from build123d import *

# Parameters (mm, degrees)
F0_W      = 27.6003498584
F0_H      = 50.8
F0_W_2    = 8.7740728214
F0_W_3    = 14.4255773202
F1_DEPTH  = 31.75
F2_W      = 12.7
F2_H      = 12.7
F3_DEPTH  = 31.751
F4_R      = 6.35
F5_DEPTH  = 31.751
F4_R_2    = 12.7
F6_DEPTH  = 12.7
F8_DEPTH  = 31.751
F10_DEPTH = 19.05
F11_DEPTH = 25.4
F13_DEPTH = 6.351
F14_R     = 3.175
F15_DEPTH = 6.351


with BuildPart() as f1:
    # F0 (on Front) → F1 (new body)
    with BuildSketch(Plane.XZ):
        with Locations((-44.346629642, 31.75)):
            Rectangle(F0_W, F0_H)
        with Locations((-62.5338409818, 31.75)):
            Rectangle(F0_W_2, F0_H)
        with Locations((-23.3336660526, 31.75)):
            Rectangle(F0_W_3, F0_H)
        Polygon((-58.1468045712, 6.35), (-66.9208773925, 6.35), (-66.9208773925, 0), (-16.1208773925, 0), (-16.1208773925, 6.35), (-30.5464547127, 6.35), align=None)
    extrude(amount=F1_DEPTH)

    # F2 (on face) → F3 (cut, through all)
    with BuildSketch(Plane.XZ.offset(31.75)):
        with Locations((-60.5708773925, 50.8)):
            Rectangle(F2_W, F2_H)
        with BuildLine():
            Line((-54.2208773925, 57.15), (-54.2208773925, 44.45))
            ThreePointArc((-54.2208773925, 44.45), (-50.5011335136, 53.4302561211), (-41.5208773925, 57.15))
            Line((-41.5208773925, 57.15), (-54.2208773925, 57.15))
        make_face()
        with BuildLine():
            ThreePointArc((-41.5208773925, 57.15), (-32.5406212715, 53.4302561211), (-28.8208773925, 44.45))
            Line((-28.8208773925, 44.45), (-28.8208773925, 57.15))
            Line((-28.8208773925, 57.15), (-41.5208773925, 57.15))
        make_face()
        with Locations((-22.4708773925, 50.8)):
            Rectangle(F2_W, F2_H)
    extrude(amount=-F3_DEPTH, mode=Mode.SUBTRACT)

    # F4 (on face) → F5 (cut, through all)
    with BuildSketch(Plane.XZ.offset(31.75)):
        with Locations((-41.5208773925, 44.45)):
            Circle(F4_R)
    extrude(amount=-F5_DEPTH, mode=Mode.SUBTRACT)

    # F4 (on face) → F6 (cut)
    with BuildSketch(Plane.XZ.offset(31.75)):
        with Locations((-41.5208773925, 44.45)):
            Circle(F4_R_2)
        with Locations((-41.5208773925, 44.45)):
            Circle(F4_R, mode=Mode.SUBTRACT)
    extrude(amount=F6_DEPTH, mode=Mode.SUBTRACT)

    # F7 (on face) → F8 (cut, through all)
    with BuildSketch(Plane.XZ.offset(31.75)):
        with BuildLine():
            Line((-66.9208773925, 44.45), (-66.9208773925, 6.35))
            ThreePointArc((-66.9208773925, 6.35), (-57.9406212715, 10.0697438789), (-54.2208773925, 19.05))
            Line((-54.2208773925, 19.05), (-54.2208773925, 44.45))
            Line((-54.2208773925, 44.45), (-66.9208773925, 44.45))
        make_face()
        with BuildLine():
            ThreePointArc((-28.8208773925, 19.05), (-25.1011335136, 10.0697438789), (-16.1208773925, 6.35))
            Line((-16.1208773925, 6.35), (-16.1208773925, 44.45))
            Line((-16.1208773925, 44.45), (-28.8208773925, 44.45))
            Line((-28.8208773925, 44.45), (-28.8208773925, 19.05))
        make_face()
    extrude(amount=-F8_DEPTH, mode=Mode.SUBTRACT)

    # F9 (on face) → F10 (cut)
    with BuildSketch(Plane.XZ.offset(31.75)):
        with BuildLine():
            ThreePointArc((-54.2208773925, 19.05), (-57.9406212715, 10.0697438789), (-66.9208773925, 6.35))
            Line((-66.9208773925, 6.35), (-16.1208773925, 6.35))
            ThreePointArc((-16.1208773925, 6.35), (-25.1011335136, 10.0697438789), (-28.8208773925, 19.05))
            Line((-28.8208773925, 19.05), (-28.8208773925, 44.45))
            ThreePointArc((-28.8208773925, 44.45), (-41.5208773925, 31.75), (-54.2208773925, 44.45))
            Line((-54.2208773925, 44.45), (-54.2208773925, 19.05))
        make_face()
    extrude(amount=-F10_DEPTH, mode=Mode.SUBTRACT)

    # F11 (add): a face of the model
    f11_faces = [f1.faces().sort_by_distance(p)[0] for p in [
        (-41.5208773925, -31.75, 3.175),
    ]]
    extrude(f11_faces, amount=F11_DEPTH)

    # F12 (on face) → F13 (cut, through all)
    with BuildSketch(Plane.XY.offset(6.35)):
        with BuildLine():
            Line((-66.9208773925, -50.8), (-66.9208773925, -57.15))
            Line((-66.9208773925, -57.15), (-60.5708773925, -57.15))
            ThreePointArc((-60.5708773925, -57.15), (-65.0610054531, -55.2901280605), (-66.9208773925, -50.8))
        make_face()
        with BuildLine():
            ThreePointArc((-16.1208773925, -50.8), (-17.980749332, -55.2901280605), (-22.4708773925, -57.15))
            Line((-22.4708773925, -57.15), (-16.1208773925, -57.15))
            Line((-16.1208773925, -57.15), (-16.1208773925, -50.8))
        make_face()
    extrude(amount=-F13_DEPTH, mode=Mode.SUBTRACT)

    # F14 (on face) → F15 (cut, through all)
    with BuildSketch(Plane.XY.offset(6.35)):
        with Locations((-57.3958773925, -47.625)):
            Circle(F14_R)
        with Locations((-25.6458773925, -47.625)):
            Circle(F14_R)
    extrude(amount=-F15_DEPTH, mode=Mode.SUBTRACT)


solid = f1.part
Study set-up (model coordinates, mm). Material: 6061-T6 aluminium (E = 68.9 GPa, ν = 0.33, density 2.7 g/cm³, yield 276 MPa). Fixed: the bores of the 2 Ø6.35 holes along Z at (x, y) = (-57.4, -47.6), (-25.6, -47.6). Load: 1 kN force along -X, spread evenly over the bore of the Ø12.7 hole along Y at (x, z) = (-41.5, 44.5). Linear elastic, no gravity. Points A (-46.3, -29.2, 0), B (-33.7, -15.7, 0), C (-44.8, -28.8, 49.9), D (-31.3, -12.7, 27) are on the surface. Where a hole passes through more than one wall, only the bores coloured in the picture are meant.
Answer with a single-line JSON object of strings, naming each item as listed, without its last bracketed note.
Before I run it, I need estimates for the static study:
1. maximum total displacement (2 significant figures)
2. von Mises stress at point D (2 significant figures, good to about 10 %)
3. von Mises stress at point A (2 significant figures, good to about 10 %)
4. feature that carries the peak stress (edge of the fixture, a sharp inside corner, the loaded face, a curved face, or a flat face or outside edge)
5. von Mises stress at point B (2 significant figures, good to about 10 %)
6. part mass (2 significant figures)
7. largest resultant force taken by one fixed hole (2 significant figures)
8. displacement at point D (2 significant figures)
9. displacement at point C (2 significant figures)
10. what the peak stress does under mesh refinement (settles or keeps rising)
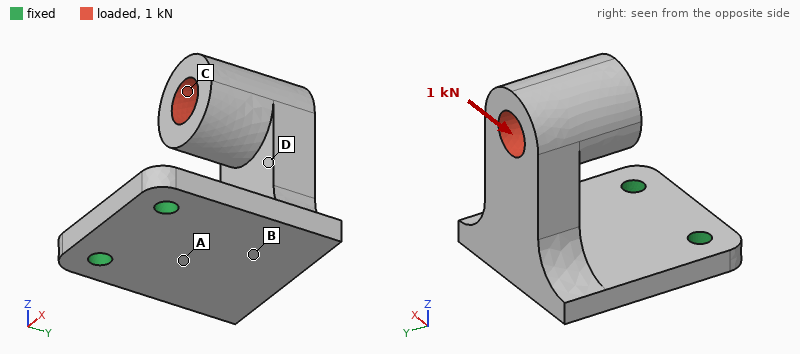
{"maximum total displacement": "0.47 mm", "von Mises stress at point D": "20 MPa", "von Mises stress at point A": "62 MPa", "feature that carries the peak stress": "edge of the fixture", "von Mises stress at point B": "54 MPa", "part mass": "110 g", "largest resultant force taken by one fixed hole": "1.5 kN", "displacement at point D": "0.21 mm", "displacement at point C": "0.41 mm", "what the peak stress does under mesh refinement": "keeps rising"}
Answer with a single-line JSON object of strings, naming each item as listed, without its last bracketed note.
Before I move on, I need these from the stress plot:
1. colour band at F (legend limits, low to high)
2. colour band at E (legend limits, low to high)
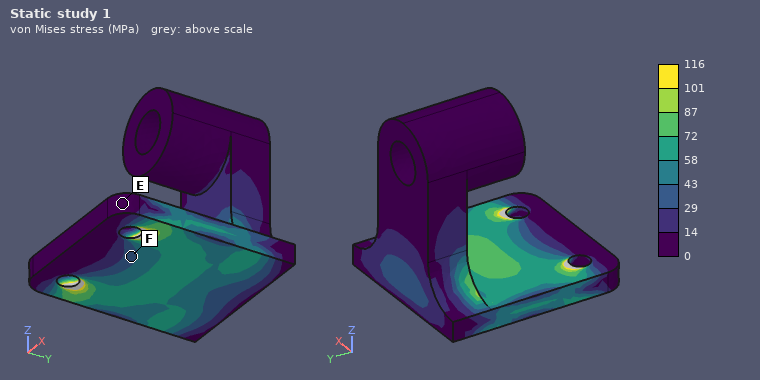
{"colour band at F": "29 to 43 MPa", "colour band at E": "0 to 14 MPa"}
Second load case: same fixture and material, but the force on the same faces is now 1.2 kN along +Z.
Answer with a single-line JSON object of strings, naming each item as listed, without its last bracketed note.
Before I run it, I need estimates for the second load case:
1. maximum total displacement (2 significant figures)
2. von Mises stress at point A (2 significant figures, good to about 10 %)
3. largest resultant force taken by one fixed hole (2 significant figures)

{"maximum total displacement": "0.45 mm", "von Mises stress at point A": "42 MPa", "largest resultant force taken by one fixed hole": "600 N"}
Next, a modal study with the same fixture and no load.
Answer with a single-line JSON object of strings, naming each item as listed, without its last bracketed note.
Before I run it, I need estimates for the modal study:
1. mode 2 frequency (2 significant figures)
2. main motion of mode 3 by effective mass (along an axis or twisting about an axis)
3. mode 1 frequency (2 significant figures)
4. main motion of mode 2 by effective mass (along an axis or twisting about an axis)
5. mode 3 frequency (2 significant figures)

{"mode 2 frequency": "1300 Hz", "main motion of mode 3 by effective mass": "along Z", "mode 1 frequency": "720 Hz", "main motion of mode 2 by effective mass": "along X", "mode 3 frequency": "2200 Hz"}
